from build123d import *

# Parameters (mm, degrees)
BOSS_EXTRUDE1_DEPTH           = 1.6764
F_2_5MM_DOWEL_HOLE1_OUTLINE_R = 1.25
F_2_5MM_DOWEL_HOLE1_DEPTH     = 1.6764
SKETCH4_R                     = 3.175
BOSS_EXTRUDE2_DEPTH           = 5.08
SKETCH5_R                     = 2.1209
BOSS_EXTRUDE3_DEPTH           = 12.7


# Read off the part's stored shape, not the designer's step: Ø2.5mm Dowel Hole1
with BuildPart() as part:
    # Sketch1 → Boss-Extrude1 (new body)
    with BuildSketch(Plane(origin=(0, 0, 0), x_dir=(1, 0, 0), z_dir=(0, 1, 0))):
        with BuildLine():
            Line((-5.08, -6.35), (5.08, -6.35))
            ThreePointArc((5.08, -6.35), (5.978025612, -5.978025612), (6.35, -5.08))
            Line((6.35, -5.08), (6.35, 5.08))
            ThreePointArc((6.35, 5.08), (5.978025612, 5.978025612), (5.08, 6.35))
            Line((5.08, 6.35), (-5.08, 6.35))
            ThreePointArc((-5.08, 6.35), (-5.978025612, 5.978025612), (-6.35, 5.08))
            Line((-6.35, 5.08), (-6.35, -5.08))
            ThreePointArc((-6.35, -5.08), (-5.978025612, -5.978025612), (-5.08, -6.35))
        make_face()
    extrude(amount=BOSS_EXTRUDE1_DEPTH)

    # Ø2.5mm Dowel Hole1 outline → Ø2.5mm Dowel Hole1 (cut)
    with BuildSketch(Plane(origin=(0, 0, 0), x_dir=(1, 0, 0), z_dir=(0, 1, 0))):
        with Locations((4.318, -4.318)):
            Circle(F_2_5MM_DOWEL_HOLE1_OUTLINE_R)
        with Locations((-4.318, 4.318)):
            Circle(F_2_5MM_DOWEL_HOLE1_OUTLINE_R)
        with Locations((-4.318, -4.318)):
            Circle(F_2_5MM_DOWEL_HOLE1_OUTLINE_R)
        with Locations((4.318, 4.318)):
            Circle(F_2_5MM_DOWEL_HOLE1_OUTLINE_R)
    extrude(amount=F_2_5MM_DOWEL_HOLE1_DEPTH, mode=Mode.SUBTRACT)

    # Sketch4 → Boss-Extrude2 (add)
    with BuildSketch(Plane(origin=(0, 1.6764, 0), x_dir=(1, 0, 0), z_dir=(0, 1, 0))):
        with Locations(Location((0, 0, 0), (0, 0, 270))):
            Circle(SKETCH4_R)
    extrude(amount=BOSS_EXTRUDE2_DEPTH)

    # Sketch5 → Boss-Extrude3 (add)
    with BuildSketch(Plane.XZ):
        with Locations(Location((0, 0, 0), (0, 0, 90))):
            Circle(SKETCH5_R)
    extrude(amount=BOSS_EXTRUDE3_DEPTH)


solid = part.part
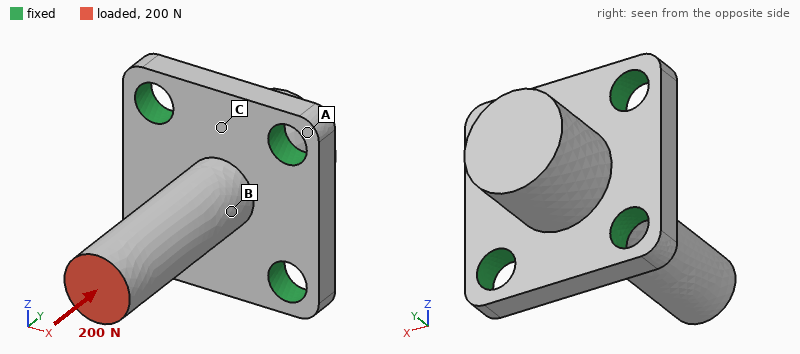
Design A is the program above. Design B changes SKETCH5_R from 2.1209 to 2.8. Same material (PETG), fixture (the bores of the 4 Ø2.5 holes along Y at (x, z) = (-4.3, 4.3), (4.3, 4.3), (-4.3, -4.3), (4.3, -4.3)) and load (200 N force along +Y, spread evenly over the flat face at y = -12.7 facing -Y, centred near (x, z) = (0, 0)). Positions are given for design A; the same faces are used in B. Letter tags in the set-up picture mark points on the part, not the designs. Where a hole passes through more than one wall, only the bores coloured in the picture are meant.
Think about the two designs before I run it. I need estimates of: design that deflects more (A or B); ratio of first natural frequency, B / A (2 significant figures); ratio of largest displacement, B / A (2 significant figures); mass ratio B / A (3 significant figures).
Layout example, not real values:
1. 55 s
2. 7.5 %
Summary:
1. A
2. 1.1
3. 0.66
4. 1.23
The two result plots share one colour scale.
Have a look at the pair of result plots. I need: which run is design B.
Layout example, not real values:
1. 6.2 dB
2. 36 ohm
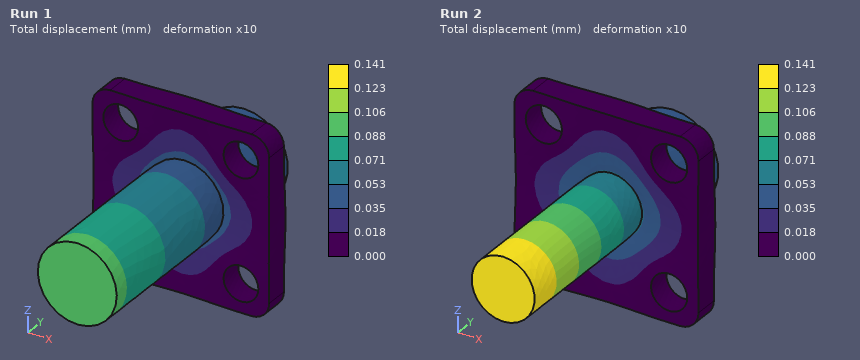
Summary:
1. Run 1
